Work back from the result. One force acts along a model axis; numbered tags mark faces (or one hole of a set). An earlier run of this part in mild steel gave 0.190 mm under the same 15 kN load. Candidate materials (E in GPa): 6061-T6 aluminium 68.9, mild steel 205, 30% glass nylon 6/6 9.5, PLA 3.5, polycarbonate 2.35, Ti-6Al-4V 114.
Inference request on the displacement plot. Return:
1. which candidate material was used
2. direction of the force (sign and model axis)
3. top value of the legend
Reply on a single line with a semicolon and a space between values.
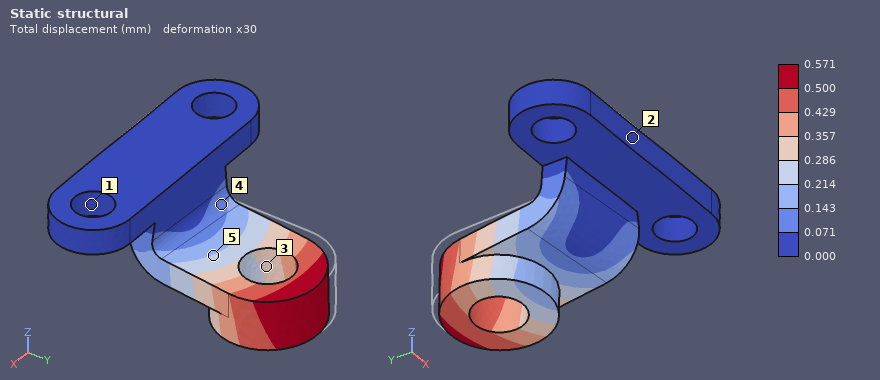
6061-T6 aluminium; +X; 0.571 mm
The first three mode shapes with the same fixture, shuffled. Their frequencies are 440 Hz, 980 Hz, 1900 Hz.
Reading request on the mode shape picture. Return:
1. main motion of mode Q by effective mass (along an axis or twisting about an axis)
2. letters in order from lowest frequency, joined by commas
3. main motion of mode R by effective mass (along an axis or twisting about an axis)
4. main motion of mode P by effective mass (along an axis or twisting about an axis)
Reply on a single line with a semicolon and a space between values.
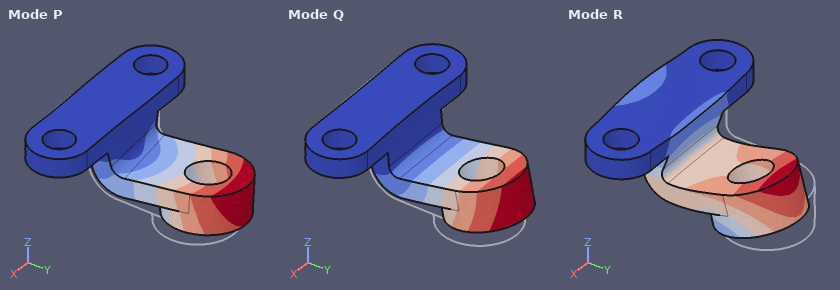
along Z; Q, P, R; along Y; along X
